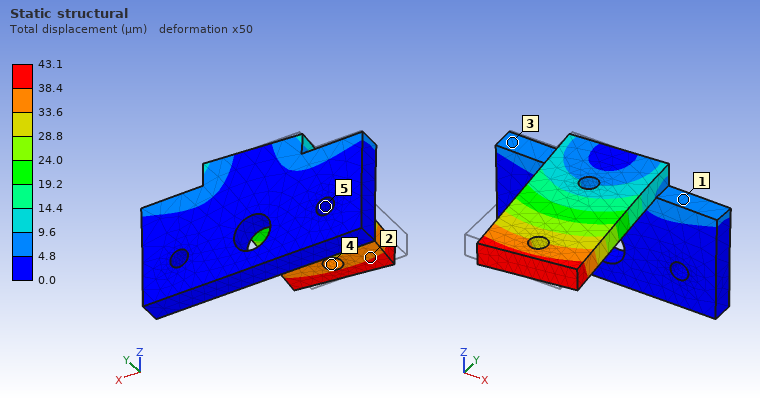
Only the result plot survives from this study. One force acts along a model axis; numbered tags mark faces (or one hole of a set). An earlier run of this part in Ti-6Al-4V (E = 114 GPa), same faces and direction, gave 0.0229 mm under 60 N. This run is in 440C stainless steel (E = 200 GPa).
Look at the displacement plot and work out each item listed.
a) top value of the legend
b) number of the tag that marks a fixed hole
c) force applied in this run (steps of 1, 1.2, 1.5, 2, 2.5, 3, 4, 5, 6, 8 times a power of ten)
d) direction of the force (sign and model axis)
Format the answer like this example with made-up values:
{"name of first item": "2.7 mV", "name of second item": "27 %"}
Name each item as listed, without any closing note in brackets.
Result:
{"top value of the legend": "43.1 µm", "number of the tag that marks a fixed hole": "5", "force applied in this run": "200 N", "direction of the force": "+X"}
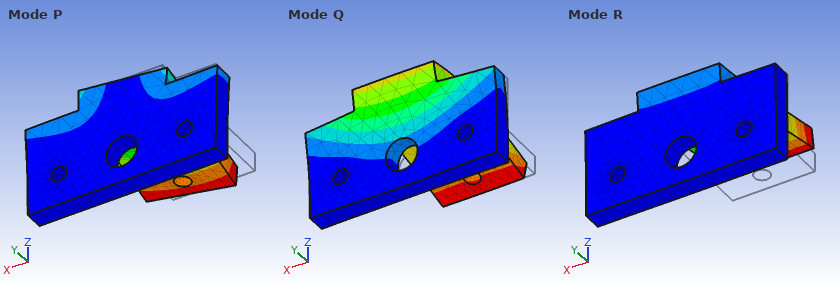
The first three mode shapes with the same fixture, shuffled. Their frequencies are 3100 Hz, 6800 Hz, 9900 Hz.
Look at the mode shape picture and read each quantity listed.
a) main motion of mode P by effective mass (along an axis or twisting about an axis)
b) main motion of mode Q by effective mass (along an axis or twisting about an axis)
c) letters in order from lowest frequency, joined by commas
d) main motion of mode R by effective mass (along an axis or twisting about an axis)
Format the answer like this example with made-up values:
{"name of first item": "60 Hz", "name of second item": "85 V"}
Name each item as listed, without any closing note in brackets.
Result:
{"main motion of mode P by effective mass": "along X", "main motion of mode Q by effective mass": "along Y", "letters in order from lowest frequency, joined by commas": "R, P, Q", "main motion of mode R by effective mass": "along Z"}
